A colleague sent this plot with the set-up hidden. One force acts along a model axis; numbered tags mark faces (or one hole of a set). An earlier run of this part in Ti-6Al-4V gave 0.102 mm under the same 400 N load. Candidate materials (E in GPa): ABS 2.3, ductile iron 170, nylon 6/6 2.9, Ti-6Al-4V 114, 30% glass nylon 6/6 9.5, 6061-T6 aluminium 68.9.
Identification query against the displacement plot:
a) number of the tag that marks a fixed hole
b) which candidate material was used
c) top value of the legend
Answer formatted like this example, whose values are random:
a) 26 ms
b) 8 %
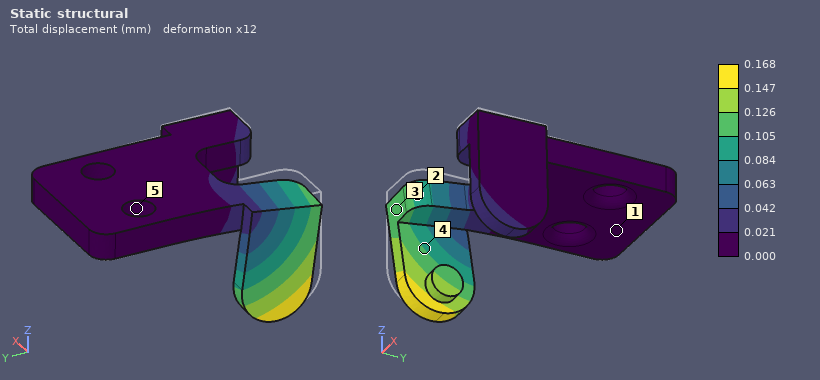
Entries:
a) 5
b) 6061-T6 aluminium
c) 0.168 mm
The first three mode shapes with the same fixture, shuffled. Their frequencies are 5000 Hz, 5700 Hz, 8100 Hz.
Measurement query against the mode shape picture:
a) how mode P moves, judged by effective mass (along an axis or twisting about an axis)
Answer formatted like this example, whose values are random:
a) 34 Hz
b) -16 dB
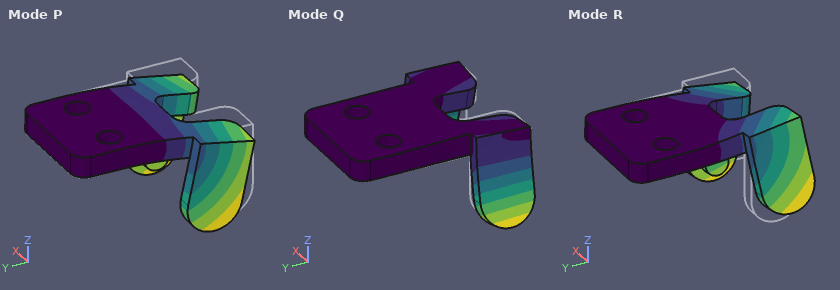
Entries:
a) along Z
